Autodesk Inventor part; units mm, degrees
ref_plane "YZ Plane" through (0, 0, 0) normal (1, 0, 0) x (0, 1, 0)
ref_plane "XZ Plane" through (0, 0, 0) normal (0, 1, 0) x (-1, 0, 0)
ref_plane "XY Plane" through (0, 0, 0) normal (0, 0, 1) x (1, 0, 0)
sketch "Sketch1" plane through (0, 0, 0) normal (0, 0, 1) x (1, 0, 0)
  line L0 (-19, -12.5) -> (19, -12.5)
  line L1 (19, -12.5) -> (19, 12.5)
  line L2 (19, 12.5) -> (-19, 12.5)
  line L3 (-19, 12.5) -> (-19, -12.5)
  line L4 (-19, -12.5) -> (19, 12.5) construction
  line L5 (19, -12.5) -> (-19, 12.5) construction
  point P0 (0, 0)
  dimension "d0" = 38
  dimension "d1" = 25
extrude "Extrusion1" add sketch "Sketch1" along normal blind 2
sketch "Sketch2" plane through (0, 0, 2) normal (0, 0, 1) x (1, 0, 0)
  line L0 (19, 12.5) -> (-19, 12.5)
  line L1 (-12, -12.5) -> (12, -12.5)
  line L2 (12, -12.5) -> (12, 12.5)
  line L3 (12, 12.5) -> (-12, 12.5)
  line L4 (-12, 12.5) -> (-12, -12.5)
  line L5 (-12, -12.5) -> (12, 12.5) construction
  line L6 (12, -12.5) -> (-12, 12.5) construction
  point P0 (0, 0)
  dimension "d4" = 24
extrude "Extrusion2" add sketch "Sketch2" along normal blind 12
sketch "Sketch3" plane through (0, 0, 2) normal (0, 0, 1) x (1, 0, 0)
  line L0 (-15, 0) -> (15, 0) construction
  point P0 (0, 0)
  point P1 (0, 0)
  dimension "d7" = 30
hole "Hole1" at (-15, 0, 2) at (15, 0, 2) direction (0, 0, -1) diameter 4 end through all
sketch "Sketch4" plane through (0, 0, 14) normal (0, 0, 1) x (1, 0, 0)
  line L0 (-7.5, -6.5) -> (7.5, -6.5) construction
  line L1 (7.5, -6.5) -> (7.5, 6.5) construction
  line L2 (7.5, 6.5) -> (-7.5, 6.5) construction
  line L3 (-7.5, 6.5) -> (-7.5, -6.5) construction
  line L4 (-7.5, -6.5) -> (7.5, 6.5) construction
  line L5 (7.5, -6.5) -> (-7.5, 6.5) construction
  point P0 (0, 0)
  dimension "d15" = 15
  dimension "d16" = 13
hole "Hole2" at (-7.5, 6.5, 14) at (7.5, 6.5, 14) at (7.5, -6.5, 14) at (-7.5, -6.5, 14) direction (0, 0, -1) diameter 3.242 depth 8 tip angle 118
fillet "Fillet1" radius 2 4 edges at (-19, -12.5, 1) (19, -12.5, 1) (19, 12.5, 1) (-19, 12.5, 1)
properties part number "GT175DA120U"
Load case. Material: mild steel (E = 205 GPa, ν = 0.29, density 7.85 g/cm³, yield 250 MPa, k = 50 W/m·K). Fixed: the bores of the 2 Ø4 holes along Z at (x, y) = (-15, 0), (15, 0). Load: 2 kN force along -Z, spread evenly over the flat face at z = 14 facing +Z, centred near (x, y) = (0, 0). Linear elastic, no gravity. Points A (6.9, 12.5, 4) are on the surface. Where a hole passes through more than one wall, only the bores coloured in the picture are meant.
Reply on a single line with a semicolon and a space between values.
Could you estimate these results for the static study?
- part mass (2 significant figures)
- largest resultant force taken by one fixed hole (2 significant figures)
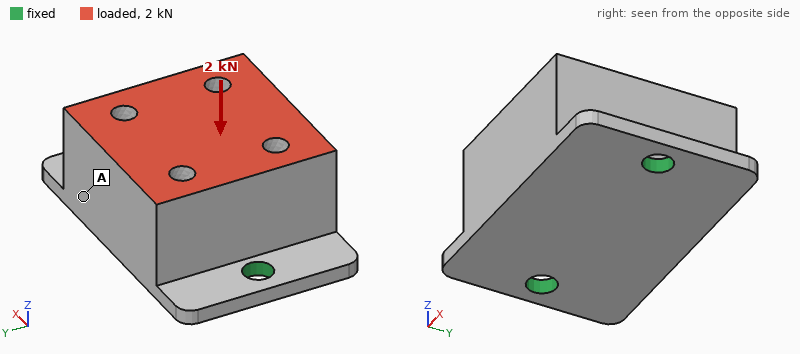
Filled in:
69 g; 1.1 kN
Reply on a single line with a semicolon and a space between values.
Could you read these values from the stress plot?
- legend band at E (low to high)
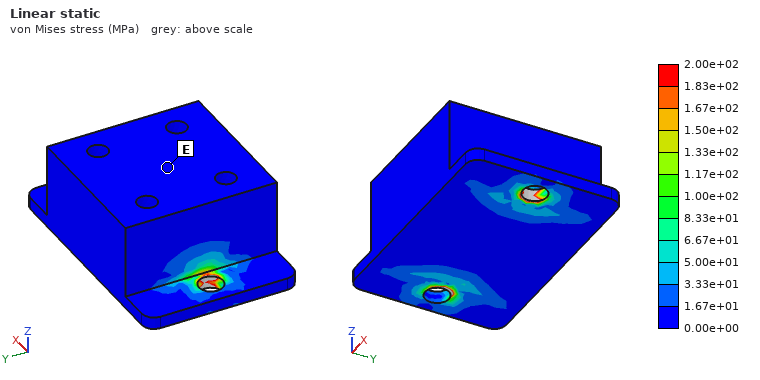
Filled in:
0.00e+00 to 1.67e+01 MPa
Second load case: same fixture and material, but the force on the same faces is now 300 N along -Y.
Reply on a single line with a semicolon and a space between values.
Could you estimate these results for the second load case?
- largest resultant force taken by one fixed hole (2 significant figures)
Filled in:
150 N
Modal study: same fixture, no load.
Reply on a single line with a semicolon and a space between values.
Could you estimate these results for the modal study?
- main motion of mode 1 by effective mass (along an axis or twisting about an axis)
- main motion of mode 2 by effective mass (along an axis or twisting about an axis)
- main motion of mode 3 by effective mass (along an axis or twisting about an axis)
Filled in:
along Y; along Z; along X
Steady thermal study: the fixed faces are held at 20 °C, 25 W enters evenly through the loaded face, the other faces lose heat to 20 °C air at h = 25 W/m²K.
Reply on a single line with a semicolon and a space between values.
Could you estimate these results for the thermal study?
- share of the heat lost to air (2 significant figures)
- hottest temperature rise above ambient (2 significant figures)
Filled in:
9.7 %; 45 K
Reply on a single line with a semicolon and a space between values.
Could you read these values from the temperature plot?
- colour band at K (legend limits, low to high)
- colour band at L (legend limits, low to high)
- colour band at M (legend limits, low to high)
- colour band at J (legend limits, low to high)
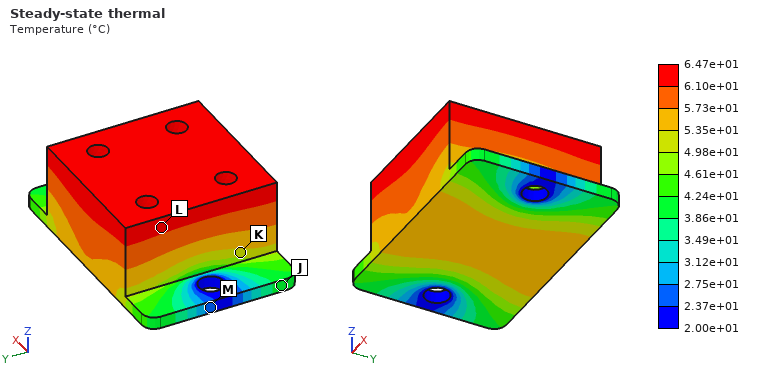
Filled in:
4.98e+01 to 5.35e+01 °C; 6.10e+01 to 6.47e+01 °C; 2.37e+01 to 2.75e+01 °C; 3.86e+01 to 4.24e+01 °C
